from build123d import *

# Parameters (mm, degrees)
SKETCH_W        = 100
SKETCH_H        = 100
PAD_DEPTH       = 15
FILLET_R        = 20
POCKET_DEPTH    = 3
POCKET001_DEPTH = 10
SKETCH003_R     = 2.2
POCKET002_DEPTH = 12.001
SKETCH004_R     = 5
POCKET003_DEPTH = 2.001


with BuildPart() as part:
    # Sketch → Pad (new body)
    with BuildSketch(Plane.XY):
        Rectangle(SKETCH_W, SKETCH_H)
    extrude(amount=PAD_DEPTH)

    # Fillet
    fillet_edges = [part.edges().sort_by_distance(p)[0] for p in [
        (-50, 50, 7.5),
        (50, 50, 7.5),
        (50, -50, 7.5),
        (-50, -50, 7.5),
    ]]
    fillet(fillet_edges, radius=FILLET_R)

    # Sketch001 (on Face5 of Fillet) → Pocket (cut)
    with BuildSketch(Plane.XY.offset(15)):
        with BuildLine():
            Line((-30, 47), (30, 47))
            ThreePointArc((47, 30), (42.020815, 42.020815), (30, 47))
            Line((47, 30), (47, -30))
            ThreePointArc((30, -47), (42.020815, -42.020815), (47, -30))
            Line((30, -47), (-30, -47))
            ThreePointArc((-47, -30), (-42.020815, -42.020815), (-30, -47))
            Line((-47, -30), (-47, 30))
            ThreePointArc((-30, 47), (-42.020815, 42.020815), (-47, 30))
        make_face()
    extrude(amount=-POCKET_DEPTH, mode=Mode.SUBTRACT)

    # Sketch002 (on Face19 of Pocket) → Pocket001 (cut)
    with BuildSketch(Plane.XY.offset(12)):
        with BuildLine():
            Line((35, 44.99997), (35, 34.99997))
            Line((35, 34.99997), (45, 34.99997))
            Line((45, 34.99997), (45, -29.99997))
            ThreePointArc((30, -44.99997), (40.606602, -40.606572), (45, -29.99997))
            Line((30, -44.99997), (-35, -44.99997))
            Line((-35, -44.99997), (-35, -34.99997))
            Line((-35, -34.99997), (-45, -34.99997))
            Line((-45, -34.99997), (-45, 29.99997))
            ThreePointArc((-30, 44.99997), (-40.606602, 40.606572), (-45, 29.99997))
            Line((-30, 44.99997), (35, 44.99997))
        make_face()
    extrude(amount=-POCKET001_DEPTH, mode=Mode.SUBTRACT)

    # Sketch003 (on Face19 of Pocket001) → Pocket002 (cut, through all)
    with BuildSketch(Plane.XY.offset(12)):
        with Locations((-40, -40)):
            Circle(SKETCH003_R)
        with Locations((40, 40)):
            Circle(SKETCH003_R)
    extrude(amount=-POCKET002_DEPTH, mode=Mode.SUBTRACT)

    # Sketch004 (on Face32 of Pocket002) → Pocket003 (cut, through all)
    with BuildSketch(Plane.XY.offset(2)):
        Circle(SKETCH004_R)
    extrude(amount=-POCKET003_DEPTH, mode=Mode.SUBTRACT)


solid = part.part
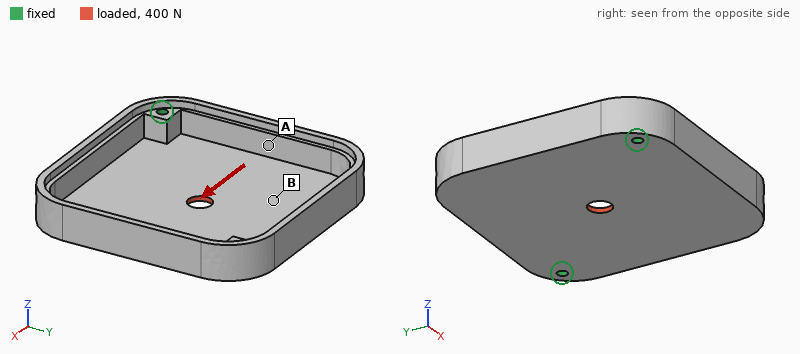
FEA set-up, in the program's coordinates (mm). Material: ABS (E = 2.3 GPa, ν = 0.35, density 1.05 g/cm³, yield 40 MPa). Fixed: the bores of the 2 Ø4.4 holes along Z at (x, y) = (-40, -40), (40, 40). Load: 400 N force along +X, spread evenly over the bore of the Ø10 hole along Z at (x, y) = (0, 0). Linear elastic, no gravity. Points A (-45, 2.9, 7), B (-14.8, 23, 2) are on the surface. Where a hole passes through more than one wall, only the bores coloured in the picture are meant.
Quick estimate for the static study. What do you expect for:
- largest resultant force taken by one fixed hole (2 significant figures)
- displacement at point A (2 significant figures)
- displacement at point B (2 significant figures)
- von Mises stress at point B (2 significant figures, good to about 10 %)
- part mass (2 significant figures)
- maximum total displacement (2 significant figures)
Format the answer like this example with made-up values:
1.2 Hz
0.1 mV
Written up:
200 N
0.071 mm
0.083 mm
2.2 MPa
43 g
0.23 mm
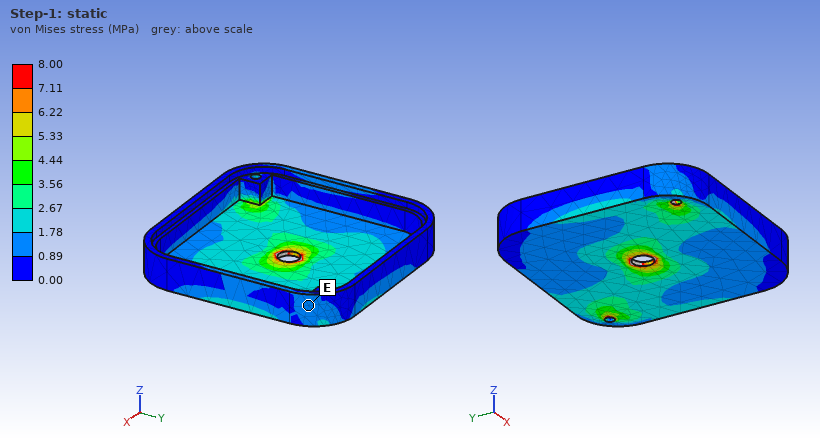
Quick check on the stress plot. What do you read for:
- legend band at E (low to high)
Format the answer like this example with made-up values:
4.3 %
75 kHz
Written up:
0.89 to 1.78 MPa
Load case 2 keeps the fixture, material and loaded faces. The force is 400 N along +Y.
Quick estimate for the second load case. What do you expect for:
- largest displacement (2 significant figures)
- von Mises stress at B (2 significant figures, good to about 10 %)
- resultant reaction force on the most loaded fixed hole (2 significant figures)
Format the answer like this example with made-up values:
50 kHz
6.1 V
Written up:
0.23 mm
2.3 MPa
200 N
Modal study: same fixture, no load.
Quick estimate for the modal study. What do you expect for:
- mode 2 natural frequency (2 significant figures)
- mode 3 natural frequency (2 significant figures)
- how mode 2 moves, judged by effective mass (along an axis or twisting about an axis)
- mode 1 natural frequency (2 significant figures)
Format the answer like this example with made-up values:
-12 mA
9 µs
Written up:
470 Hz
650 Hz
along Z
450 Hz
